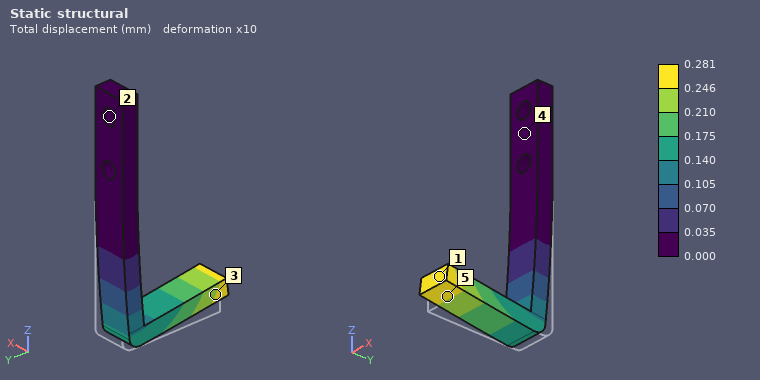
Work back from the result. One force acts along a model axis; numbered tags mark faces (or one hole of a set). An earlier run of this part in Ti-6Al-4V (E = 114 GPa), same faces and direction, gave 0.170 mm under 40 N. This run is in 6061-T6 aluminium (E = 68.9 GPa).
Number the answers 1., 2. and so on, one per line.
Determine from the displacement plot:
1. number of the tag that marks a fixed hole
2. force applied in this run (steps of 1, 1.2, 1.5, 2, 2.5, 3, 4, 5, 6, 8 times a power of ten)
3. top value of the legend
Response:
1. 2
2. 40 N
3. 0.281 mm
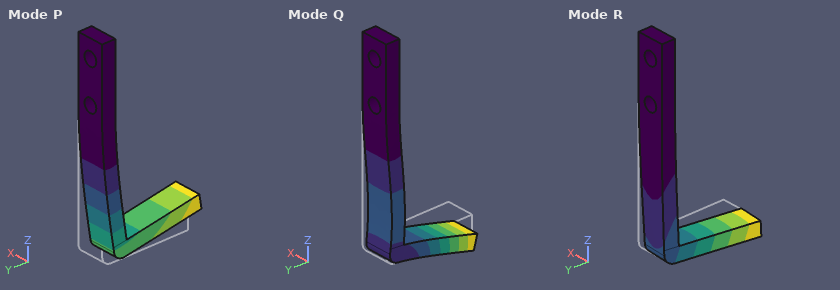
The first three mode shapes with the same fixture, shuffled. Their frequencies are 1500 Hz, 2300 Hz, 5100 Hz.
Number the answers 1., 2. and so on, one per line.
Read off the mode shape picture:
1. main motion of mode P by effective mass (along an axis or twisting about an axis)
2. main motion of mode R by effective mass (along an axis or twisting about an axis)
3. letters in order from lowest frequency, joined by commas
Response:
1. along Y
2. along X
3. P, R, Q
